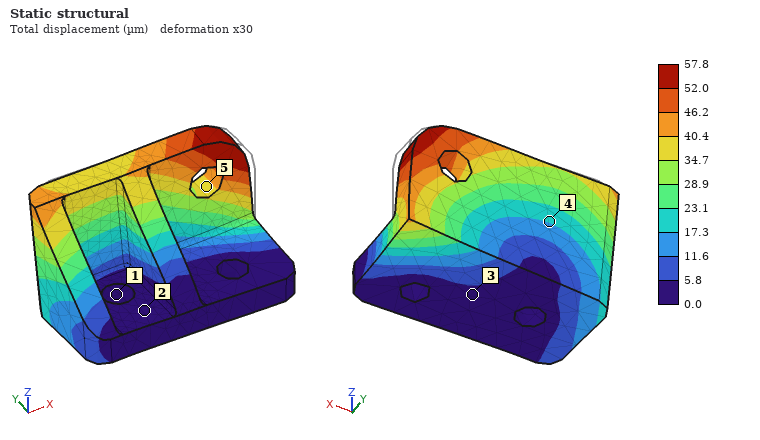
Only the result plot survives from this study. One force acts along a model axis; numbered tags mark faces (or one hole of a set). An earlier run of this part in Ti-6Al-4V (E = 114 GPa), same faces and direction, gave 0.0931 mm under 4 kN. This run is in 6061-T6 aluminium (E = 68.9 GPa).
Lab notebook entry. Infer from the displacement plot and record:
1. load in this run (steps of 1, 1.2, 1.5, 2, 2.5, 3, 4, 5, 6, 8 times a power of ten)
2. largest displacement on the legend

1.5 kN
57.8 µm
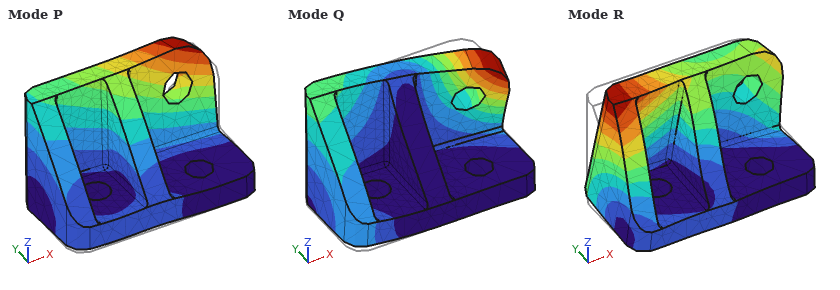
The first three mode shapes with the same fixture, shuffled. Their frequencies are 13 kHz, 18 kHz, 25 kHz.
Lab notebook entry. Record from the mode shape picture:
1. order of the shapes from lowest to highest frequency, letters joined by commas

P, R, Q
